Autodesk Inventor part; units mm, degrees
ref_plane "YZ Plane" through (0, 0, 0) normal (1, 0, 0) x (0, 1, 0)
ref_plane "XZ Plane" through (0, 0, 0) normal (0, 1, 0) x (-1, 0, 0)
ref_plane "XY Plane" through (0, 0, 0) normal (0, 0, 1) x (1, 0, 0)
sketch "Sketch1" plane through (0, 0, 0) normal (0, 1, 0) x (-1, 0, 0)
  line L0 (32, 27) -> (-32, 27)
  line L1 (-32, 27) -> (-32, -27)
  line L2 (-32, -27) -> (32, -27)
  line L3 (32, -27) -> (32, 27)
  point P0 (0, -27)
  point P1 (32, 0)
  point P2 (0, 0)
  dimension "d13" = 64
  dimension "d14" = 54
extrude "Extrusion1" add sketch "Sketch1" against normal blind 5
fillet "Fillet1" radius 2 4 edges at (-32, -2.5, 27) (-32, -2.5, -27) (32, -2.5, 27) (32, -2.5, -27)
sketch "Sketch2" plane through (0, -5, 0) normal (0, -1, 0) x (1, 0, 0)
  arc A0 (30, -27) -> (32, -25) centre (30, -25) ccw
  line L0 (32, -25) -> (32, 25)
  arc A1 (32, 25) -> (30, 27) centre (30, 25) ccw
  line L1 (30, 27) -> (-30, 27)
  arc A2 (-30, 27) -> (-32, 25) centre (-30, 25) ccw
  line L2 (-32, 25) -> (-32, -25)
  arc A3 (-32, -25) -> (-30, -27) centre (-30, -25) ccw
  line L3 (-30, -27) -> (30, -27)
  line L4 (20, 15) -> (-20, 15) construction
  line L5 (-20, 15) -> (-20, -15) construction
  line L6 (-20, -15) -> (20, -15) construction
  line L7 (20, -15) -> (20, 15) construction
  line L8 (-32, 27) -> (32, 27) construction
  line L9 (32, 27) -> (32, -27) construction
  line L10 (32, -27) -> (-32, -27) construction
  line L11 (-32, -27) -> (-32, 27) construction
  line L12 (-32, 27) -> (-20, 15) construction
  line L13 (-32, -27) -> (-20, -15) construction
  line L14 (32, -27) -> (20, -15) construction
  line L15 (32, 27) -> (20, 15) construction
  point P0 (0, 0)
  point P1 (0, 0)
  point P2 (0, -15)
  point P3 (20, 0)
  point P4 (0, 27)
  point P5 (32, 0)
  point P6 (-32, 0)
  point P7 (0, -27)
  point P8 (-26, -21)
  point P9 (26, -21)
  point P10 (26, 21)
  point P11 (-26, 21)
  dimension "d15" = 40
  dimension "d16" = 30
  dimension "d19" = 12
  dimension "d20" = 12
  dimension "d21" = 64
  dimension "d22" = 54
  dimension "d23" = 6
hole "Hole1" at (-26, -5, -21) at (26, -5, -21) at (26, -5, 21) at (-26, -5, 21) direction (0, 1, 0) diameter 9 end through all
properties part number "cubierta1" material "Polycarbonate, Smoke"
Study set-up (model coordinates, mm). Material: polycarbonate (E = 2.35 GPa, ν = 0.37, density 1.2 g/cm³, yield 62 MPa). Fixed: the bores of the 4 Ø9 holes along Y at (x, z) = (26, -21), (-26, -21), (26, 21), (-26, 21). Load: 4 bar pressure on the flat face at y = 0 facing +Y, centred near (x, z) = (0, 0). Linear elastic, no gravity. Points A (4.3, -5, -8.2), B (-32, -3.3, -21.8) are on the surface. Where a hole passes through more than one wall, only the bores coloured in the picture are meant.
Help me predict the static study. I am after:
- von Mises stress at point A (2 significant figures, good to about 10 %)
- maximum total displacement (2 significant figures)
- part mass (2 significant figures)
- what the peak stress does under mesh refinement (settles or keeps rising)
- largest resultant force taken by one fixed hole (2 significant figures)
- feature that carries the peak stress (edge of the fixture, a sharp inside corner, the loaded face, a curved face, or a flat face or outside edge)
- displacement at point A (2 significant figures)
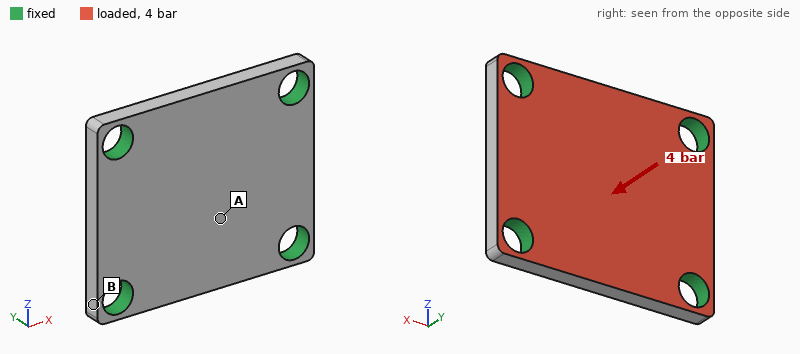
8.3 MPa
0.35 mm
19 g
keeps rising
320 N
edge of the fixture
0.32 mm
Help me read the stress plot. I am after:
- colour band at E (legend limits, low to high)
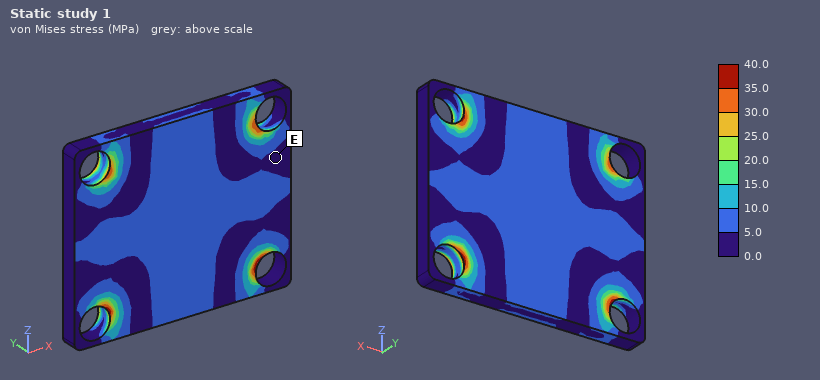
0.0 to 5.0 MPa
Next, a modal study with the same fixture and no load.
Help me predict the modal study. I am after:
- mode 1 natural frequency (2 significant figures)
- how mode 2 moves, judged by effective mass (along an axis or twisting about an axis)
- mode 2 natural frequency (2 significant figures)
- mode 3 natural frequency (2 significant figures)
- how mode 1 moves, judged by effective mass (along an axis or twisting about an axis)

2600 Hz
twisting about X
3700 Hz
4600 Hz
along Y
